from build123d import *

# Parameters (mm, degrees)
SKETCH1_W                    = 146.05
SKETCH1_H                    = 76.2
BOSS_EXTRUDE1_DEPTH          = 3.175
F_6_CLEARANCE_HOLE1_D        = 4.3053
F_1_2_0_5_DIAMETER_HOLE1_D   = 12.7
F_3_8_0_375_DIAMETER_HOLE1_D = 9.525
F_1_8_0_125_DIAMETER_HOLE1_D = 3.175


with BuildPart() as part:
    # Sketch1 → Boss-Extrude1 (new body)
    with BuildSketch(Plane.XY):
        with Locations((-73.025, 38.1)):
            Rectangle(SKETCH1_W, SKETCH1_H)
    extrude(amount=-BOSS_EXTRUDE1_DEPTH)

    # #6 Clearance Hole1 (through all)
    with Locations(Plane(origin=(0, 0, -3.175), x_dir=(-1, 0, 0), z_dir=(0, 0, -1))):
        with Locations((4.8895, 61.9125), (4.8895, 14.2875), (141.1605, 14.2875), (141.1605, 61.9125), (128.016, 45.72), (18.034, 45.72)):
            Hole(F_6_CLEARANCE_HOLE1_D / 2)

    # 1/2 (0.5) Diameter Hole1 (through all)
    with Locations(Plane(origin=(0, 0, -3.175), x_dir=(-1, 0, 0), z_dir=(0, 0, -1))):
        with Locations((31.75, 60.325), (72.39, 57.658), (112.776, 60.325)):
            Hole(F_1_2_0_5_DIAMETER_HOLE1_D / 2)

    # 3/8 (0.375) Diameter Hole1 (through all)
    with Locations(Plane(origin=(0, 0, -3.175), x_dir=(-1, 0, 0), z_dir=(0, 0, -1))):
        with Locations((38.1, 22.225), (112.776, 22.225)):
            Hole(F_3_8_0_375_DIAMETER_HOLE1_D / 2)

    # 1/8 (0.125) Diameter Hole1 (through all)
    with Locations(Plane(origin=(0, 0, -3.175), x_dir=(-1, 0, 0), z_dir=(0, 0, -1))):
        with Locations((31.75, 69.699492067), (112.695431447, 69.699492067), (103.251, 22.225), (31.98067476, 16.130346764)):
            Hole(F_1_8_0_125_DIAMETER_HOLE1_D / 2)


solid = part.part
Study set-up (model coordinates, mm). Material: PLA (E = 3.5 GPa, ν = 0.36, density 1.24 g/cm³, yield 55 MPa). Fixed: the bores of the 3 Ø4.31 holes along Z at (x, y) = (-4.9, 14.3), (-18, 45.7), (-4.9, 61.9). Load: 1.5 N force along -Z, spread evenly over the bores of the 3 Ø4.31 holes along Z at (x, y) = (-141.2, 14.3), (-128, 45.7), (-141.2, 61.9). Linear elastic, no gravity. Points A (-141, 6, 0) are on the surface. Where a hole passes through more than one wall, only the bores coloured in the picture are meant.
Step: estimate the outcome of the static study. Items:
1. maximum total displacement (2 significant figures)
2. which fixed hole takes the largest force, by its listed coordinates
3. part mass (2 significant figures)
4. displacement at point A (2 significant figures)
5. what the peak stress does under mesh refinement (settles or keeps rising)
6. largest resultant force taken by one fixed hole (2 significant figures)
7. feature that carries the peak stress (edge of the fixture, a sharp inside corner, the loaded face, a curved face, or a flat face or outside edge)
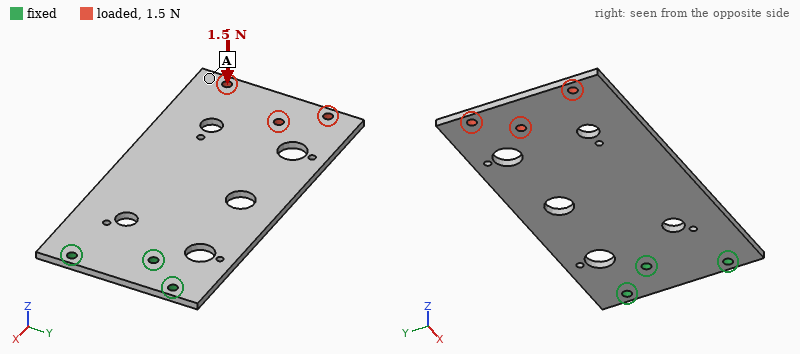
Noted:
1.6 mm
(-18, 45.7)
41 g
1.5 mm
keeps rising
5.9 N
edge of the fixture
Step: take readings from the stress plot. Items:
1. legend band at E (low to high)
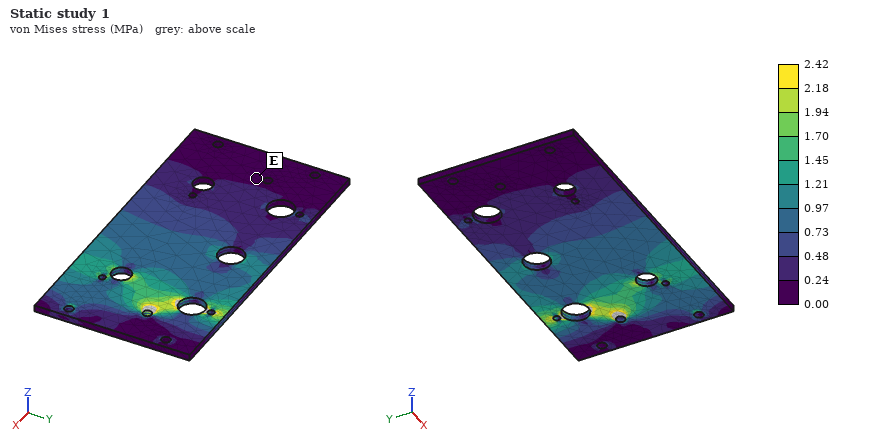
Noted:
0.00 to 0.24 MPa
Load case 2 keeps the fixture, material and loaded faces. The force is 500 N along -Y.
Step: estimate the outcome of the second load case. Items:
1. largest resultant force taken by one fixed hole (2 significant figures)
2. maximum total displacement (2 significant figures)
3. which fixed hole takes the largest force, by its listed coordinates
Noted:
1.2 kN
1.9 mm
(-4.9, 14.3)
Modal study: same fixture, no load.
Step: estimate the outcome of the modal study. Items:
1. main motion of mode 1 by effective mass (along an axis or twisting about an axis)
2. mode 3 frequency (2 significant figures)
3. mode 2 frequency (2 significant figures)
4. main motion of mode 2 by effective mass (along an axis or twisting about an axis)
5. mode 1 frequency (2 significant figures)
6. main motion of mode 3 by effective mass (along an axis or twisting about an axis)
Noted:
along Z
300 Hz
170 Hz
twisting about X
49 Hz
along Z
